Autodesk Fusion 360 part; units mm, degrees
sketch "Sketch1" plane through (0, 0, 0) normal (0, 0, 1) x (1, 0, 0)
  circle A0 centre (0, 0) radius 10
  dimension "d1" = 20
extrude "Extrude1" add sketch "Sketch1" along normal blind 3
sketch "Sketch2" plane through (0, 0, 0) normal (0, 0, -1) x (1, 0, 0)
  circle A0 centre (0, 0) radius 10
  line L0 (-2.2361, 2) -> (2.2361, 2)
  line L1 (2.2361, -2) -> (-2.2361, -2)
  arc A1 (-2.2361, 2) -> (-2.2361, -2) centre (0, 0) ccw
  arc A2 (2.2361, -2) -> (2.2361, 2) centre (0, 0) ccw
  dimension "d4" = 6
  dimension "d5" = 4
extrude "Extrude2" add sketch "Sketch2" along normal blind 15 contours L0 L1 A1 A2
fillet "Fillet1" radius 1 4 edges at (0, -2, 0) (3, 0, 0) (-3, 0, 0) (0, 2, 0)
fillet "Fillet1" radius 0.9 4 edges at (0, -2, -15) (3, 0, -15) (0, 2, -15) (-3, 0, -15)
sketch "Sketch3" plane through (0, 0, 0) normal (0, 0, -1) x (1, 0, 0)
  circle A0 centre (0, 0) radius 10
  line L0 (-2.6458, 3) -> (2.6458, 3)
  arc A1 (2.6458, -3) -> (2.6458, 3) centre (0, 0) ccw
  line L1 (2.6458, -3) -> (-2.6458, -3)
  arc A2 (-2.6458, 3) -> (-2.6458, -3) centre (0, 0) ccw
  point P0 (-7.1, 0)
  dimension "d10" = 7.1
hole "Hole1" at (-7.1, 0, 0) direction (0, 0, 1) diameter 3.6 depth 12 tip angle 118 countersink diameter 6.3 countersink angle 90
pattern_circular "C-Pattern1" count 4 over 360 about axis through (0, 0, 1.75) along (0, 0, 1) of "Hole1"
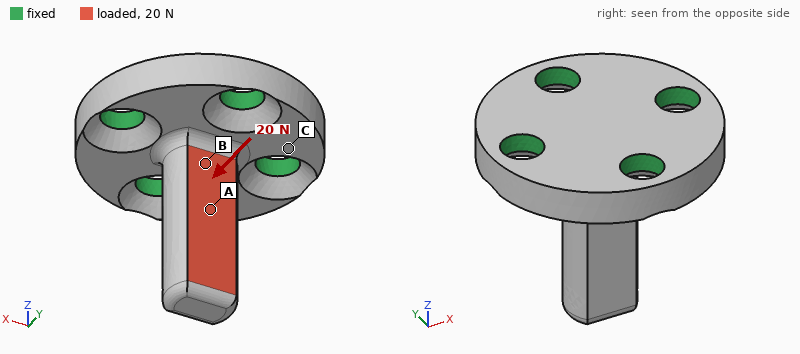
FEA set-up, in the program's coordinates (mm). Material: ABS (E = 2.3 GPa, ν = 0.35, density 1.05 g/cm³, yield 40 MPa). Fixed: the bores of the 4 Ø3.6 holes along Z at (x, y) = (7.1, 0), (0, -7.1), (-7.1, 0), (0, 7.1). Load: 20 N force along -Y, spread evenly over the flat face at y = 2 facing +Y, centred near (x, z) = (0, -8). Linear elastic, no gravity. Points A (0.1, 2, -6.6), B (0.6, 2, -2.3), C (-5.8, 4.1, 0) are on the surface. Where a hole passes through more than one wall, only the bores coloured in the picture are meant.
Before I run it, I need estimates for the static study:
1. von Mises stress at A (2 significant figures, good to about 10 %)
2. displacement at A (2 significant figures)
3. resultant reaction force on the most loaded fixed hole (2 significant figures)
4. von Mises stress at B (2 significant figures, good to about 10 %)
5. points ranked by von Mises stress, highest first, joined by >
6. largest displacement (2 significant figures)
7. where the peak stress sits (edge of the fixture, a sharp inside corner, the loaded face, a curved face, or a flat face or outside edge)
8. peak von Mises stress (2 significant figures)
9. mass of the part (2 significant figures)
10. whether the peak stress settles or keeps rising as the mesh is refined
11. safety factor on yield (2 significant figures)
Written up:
3.4 MPa
0.064 mm
18 N
7.5 MPa
B > A > C
0.17 mm
a curved face
15 MPa
1.2 g
settles
2.6
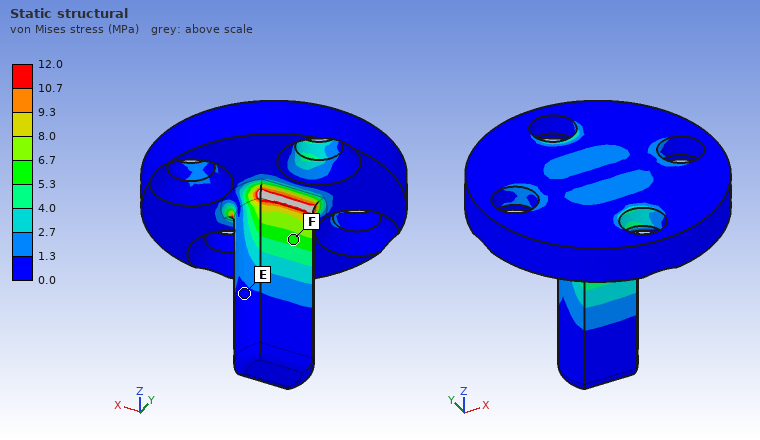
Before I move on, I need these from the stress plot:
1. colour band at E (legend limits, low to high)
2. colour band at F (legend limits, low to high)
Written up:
0.0 to 1.3 MPa
5.3 to 6.7 MPa
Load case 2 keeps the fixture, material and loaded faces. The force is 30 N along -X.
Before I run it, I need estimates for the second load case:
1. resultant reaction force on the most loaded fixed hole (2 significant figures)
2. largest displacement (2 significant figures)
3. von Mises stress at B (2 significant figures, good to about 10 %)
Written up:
28 N
0.15 mm
6.9 MPa
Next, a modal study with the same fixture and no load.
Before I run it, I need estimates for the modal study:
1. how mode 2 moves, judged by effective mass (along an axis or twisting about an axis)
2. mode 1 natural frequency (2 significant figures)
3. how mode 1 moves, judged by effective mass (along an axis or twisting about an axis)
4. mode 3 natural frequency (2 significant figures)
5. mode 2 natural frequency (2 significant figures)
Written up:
along X
3600 Hz
along Y
14 kHz
4800 Hz
